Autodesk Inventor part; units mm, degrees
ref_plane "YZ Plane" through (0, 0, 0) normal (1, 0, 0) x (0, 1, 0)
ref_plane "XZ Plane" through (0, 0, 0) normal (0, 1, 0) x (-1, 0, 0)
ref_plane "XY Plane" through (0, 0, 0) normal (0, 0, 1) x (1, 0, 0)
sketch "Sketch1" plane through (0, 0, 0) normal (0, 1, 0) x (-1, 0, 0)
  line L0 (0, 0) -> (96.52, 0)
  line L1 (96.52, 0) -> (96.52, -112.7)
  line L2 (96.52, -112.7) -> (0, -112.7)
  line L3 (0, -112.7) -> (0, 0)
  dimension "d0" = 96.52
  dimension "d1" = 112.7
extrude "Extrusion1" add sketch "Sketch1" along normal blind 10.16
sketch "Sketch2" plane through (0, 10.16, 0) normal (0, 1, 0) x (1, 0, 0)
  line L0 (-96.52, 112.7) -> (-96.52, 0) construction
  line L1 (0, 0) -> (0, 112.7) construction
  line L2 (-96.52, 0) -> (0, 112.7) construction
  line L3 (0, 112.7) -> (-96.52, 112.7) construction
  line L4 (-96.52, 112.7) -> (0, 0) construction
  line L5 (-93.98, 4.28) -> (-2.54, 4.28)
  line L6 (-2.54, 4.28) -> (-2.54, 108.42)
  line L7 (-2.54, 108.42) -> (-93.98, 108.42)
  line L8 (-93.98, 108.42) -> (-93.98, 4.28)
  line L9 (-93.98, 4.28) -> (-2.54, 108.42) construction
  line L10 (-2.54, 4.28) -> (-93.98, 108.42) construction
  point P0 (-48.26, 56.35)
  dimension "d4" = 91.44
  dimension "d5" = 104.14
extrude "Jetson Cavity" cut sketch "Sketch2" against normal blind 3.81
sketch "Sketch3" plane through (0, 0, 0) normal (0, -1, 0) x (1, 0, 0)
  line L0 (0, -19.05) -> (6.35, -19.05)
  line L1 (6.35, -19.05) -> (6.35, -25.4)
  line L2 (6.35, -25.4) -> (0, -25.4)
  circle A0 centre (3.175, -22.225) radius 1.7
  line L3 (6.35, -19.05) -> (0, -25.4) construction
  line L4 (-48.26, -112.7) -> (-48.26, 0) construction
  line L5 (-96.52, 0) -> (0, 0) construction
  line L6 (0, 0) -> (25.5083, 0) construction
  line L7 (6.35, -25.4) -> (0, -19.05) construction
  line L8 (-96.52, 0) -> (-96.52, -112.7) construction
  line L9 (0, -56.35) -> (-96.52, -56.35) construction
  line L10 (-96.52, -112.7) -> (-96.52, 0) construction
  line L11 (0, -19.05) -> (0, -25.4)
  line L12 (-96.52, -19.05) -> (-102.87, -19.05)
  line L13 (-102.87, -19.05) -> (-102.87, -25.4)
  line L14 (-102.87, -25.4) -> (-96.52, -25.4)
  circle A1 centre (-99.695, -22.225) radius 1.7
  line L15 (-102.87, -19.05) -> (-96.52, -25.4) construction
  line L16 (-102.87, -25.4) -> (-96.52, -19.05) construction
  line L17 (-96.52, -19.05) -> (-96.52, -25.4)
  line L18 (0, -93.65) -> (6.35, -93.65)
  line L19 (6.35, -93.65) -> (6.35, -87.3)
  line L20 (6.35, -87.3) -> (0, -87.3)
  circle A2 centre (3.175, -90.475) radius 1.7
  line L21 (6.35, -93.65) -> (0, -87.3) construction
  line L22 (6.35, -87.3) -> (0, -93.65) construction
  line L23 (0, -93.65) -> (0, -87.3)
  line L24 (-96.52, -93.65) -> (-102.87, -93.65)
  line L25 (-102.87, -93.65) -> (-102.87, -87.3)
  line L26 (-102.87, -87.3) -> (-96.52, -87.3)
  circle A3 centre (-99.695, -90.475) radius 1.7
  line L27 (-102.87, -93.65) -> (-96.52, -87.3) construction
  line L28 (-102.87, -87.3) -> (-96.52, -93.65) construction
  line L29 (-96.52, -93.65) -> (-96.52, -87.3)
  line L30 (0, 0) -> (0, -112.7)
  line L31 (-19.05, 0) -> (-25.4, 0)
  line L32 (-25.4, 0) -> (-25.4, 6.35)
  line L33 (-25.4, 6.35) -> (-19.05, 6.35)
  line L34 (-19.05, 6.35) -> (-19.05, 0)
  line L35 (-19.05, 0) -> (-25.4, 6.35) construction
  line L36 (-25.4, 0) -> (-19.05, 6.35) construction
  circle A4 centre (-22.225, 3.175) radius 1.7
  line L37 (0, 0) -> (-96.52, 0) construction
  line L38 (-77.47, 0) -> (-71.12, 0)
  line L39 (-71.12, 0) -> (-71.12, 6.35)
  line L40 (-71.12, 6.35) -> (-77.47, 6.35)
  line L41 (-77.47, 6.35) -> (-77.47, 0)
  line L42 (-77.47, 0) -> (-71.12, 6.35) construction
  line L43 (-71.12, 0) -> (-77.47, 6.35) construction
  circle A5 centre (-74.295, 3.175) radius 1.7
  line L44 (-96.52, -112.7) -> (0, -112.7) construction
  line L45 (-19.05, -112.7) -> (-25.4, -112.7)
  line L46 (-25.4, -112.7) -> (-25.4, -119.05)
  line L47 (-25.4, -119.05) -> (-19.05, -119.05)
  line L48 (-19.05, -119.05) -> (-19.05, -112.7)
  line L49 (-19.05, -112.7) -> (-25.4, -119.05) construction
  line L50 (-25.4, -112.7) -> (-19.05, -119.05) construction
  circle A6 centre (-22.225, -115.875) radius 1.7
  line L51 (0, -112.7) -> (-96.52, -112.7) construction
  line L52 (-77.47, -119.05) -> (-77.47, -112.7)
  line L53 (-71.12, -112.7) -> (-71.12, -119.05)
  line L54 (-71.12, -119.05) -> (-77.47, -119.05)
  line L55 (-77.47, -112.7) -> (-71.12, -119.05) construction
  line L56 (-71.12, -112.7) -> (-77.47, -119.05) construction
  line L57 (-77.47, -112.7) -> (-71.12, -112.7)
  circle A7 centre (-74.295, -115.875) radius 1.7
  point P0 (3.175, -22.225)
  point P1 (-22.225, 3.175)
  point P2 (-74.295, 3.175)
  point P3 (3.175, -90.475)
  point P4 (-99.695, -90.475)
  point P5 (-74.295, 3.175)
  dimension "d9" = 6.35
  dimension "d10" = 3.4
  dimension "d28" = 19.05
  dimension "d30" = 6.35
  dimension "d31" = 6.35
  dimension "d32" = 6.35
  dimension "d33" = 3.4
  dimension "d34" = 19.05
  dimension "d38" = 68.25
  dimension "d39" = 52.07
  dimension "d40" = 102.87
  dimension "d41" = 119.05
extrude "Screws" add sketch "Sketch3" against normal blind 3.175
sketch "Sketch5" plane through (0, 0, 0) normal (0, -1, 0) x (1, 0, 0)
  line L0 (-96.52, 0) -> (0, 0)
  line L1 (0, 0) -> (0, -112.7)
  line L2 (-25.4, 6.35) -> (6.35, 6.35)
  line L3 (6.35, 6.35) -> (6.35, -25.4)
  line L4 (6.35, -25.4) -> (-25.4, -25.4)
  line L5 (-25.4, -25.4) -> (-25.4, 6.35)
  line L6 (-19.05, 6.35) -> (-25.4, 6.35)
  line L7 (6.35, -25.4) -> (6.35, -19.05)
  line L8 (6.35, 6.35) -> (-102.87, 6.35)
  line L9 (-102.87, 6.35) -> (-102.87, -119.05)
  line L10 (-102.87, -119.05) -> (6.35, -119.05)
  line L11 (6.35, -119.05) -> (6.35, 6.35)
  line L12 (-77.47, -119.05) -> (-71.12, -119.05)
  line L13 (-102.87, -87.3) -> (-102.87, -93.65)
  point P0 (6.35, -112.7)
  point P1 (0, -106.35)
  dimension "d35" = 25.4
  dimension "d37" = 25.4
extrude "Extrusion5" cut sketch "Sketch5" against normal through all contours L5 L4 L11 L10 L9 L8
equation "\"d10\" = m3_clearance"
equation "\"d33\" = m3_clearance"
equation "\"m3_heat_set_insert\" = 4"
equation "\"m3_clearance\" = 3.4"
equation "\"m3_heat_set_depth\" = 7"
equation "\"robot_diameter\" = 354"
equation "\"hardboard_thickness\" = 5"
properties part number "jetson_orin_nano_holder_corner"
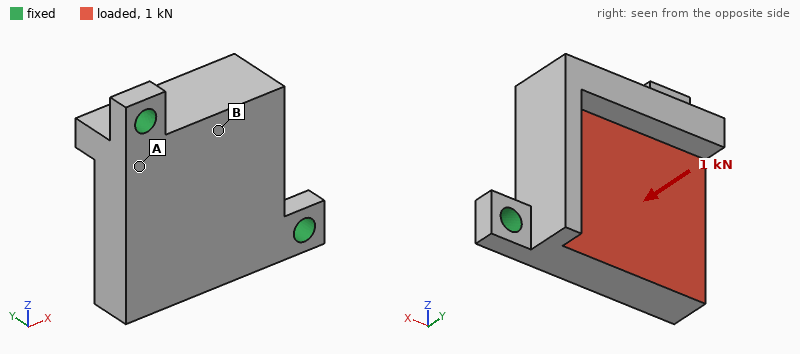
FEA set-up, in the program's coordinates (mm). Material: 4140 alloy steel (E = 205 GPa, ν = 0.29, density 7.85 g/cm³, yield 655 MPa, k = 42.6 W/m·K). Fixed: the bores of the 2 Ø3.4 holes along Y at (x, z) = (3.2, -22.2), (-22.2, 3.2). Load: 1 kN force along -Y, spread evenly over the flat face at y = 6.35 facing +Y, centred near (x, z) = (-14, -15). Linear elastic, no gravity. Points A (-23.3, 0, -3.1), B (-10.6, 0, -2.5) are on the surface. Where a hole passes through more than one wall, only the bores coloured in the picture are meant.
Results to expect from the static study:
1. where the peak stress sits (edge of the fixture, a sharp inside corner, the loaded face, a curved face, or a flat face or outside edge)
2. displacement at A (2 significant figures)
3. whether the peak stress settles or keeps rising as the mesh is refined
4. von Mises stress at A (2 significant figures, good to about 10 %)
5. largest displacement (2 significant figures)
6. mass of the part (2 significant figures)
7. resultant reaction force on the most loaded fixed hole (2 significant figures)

edge of the fixture
10.0 µm
keeps rising
53 MPa
59 µm
39 g
610 N
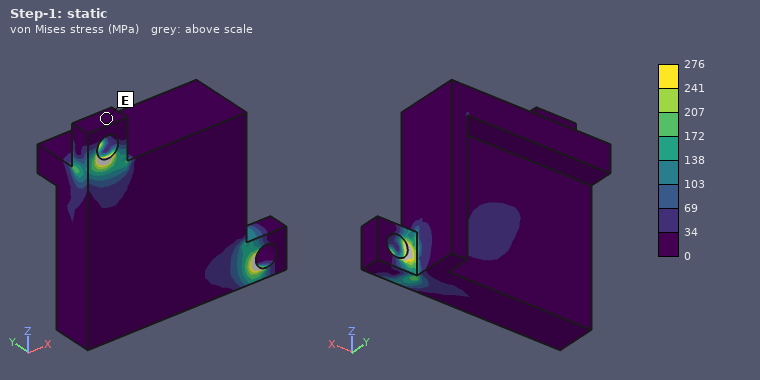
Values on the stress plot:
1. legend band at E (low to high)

0 to 34 MPa
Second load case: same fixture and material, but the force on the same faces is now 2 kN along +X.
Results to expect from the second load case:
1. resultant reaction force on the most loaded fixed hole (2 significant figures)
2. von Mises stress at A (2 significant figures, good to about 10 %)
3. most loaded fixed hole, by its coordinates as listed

1.4 kN
51 MPa
(3.2, -22.2)
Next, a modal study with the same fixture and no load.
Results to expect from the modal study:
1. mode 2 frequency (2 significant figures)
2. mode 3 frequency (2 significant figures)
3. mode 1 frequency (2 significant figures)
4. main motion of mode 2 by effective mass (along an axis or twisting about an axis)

11 kHz
20 kHz
4700 Hz
along Y
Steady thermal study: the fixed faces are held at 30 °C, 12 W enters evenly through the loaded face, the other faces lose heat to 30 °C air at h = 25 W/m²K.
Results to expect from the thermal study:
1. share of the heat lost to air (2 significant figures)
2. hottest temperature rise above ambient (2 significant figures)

12 %
41 K
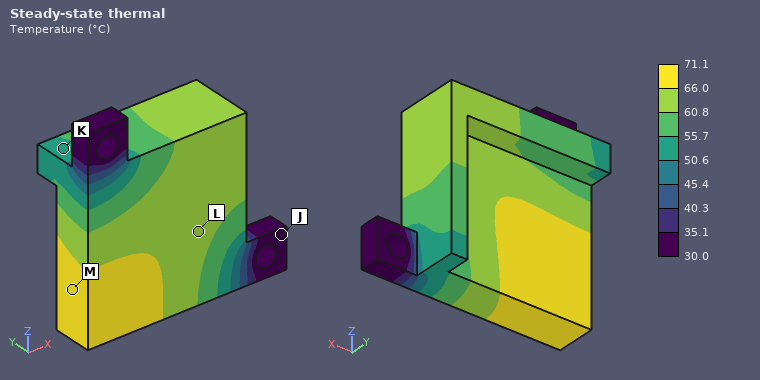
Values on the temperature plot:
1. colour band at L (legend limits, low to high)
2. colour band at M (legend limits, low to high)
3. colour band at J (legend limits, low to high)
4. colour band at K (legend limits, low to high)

60.8 to 66.0 °C
66.0 to 71.1 °C
30.0 to 35.1 °C
50.6 to 55.7 °C
